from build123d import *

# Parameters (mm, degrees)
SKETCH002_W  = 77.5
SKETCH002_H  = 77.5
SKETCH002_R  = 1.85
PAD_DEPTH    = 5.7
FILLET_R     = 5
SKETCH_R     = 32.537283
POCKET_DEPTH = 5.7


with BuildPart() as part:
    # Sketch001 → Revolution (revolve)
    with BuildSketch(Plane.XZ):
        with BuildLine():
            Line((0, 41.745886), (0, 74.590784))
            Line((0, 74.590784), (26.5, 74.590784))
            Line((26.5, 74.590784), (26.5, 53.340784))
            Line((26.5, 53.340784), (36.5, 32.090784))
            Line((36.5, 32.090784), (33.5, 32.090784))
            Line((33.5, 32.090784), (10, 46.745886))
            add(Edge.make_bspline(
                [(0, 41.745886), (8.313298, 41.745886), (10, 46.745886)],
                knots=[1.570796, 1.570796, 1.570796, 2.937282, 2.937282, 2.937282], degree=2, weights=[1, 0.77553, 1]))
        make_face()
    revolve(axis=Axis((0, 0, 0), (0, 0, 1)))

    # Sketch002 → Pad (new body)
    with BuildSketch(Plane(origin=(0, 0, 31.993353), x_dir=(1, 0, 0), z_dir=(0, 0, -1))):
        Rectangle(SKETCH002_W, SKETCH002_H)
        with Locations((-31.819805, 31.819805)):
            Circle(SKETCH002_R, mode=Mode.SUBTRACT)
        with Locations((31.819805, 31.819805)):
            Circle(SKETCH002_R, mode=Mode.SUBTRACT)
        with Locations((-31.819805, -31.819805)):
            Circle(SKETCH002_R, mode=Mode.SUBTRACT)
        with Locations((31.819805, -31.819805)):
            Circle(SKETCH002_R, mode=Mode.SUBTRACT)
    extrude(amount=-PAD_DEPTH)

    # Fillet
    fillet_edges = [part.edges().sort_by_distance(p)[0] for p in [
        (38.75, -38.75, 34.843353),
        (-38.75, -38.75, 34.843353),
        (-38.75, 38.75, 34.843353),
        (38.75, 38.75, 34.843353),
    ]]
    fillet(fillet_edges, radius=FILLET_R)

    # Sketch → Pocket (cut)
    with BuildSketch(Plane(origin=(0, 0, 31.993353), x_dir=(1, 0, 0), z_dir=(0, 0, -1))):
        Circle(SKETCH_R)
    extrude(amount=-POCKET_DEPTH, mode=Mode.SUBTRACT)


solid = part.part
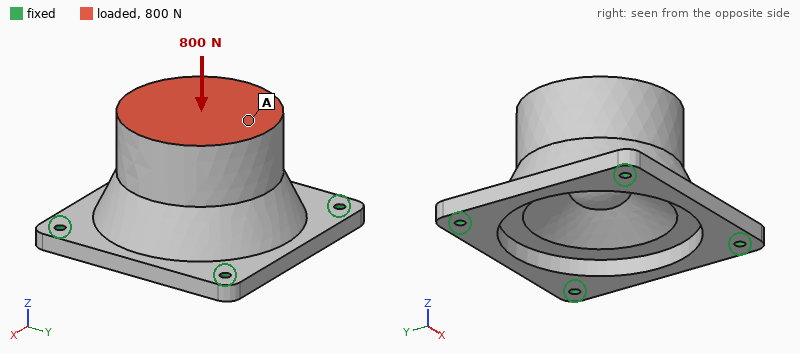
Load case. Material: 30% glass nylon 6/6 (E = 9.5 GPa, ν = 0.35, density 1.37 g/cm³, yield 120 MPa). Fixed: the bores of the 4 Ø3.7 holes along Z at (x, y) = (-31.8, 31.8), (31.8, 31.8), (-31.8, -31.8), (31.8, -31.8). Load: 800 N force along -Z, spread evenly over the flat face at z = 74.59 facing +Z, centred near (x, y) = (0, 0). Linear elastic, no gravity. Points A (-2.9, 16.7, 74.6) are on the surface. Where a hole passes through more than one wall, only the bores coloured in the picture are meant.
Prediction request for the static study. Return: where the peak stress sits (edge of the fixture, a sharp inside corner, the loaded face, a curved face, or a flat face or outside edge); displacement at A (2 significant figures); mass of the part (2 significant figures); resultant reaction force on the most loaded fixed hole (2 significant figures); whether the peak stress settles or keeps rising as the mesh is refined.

edge of the fixture
37 µm
140 g
290 N
keeps rising
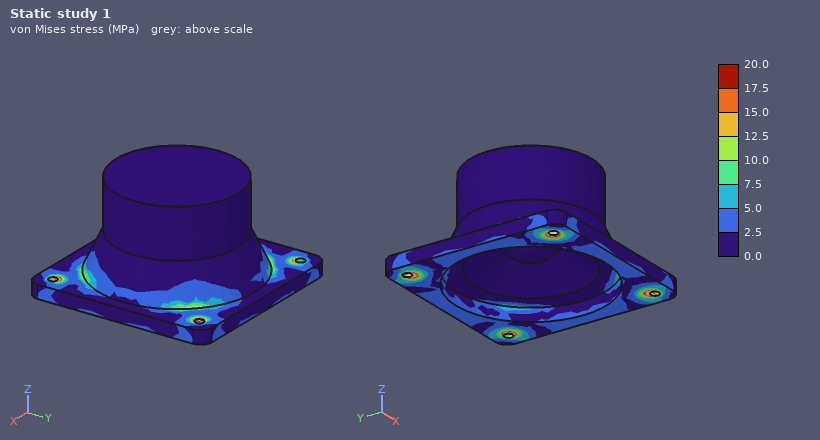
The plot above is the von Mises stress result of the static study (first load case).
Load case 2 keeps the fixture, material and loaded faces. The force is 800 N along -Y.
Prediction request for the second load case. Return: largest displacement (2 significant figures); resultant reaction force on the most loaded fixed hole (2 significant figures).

100 µm
420 N
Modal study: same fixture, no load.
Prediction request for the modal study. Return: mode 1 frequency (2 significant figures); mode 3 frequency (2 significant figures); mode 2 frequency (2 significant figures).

2100 Hz
2100 Hz
2100 Hz
